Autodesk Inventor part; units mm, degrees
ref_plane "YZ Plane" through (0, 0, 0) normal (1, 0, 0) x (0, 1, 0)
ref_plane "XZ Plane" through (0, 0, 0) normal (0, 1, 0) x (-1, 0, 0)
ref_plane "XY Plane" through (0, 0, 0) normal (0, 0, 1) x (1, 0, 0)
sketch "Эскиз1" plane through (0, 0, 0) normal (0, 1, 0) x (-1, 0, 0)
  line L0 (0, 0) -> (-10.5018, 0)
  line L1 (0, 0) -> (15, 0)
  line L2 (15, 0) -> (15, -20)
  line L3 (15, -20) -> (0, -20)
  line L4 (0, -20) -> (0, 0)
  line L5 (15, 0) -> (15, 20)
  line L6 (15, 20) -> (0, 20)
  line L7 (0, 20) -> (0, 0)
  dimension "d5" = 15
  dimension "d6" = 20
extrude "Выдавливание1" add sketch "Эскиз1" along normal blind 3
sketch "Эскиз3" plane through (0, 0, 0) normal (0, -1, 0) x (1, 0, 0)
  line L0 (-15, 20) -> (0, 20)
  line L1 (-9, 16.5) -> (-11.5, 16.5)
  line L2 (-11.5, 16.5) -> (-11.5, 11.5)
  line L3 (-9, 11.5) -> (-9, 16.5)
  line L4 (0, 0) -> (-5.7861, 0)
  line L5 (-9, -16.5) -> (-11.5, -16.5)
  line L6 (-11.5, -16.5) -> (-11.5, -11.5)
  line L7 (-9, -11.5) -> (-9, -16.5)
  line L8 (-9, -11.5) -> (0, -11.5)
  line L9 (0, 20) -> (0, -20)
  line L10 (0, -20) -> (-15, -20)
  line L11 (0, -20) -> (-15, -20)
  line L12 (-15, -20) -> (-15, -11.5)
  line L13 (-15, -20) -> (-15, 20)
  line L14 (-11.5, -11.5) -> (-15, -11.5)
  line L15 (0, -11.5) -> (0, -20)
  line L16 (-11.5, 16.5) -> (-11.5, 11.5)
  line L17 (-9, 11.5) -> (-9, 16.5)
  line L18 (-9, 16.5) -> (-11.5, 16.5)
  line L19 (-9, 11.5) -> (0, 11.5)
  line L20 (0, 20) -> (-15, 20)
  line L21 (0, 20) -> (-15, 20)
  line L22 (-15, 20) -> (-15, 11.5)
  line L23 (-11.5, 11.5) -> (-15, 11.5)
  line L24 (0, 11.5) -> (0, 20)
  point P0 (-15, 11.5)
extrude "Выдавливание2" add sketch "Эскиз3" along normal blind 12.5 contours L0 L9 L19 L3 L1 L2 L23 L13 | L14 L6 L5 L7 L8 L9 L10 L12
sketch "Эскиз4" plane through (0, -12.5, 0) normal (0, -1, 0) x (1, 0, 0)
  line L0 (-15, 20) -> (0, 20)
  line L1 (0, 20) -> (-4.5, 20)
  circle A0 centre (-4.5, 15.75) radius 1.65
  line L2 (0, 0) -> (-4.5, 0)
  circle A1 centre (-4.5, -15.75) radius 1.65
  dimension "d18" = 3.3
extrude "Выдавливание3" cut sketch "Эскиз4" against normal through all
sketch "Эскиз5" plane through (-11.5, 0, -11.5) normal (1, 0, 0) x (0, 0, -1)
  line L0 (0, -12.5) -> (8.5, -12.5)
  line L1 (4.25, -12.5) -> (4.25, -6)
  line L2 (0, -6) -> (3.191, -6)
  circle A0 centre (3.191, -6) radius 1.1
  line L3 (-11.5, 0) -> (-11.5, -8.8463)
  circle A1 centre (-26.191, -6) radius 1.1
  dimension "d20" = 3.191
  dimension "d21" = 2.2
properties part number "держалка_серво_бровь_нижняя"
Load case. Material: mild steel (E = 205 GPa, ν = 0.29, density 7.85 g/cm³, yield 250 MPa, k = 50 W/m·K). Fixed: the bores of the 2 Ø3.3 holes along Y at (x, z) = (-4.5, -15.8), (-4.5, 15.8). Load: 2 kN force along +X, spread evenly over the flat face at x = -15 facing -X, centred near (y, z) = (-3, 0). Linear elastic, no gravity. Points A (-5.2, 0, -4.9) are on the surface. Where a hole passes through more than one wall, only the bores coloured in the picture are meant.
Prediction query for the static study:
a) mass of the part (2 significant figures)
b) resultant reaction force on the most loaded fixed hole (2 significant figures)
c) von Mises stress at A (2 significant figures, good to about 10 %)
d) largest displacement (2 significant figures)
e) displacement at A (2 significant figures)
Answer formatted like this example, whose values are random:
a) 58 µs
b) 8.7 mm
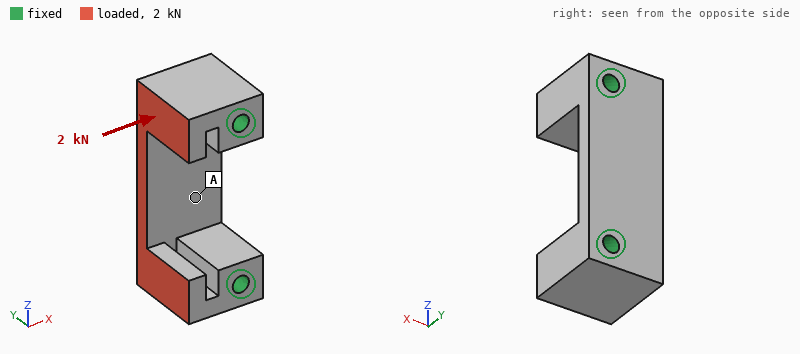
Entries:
a) 35 g
b) 1.0 kN
c) 5.6 MPa
d) 5.2 µm
e) 1.2 µm
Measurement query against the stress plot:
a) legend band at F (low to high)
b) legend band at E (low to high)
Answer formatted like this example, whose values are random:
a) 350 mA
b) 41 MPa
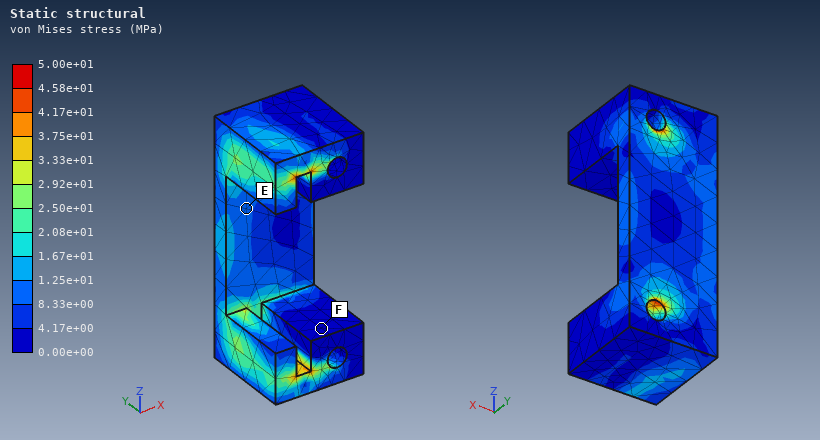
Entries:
a) 0.00e+00 to 4.17e+00 MPa
b) 8.33e+00 to 1.25e+01 MPa
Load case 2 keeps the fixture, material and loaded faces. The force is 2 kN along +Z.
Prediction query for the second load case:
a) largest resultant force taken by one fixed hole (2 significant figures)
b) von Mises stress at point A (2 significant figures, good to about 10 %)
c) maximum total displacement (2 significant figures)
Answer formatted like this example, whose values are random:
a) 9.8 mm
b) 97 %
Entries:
a) 1.1 kN
b) 12 MPa
c) 11 µm
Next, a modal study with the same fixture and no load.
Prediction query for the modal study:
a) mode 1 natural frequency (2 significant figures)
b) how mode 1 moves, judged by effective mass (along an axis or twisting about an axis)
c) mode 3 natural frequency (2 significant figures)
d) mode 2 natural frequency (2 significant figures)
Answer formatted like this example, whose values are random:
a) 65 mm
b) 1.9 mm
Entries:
a) 20 kHz
b) along Y
c) 32 kHz
d) 28 kHz
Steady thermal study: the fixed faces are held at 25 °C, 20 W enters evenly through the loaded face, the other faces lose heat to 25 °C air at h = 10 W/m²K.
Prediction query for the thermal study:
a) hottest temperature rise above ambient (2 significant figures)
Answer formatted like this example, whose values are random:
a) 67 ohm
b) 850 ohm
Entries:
a) 23 K
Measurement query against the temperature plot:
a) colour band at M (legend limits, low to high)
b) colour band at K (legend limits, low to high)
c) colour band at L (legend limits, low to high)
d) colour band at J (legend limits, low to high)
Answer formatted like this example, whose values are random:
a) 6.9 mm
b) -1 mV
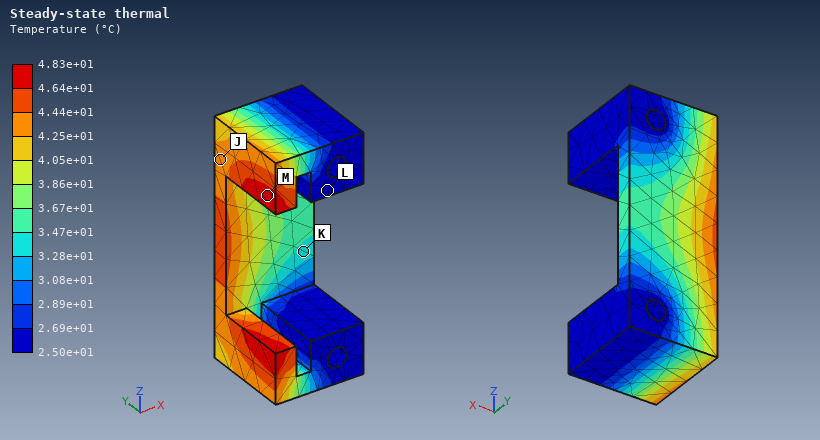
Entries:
a) 4.64e+01 to 4.83e+01 °C
b) 3.28e+01 to 3.47e+01 °C
c) 2.50e+01 to 2.69e+01 °C
d) 4.25e+01 to 4.44e+01 °C
